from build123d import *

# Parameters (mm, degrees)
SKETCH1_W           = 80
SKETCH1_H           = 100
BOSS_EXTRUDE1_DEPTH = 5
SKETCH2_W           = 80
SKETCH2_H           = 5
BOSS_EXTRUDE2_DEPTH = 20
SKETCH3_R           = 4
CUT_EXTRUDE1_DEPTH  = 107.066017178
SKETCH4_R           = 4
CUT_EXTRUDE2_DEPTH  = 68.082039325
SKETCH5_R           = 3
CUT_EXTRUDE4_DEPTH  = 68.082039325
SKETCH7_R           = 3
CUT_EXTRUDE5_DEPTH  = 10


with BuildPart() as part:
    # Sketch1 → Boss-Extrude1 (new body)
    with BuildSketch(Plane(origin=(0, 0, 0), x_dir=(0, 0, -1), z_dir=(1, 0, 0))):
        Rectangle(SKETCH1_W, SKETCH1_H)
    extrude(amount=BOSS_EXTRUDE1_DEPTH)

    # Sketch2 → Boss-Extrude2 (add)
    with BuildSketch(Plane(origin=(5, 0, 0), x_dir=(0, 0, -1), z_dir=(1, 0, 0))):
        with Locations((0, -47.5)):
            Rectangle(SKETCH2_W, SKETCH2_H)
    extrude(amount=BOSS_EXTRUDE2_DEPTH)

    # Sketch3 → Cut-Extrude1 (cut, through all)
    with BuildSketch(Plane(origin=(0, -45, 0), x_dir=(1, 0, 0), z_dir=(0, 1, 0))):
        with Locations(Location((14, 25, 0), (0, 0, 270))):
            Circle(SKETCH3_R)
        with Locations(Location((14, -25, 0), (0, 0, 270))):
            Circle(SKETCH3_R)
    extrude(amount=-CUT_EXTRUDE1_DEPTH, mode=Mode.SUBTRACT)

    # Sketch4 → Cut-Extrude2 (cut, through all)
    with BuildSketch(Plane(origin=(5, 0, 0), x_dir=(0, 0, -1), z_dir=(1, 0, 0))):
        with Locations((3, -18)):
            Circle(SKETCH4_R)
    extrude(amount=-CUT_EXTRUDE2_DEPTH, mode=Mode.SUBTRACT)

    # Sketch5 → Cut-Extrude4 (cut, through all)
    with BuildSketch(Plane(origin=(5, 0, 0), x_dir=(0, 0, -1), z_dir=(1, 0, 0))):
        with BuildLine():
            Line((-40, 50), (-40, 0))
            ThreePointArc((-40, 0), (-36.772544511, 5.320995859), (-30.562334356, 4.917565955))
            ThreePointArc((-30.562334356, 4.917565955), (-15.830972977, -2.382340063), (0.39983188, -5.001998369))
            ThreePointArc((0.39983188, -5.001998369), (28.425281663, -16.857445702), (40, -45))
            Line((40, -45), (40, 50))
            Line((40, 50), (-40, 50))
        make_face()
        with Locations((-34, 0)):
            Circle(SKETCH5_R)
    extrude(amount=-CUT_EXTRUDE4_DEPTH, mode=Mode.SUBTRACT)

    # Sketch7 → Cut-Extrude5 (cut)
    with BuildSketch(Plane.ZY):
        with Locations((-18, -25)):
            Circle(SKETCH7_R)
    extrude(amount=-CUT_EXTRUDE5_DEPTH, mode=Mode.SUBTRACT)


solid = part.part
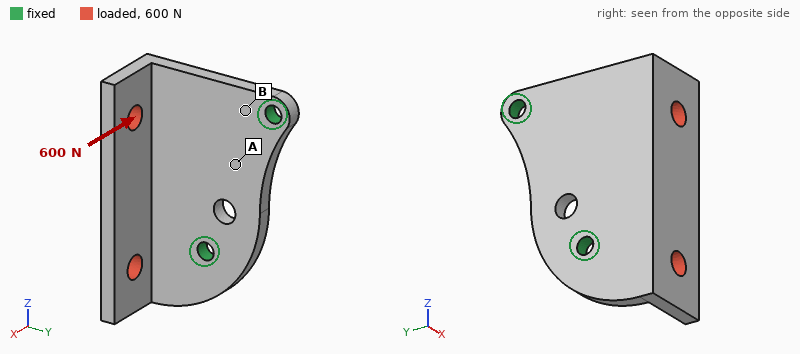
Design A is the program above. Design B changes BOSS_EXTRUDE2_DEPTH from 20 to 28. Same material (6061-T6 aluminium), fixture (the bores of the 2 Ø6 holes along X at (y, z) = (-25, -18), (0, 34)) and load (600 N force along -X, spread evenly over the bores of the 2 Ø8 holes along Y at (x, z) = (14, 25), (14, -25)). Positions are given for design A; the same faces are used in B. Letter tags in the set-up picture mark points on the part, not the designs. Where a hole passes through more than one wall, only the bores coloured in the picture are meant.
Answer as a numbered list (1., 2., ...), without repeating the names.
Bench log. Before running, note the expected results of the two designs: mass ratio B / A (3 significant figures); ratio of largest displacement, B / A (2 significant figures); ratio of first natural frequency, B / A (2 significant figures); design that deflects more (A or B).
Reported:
1. 1.13
2. 1.1
3. 0.83
4. B
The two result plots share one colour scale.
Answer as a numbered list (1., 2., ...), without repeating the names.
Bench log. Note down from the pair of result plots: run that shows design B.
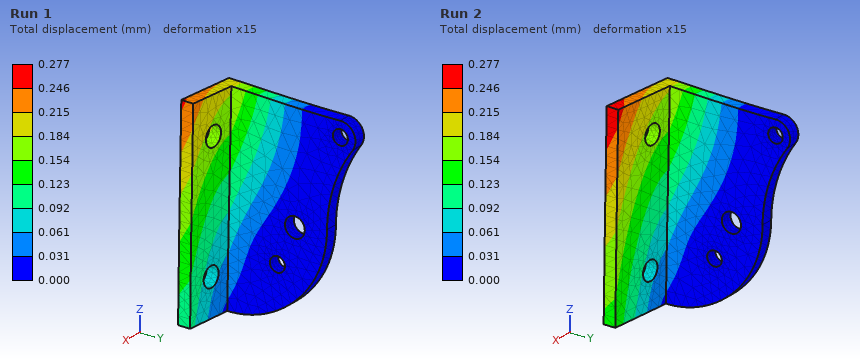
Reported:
1. Run 2
